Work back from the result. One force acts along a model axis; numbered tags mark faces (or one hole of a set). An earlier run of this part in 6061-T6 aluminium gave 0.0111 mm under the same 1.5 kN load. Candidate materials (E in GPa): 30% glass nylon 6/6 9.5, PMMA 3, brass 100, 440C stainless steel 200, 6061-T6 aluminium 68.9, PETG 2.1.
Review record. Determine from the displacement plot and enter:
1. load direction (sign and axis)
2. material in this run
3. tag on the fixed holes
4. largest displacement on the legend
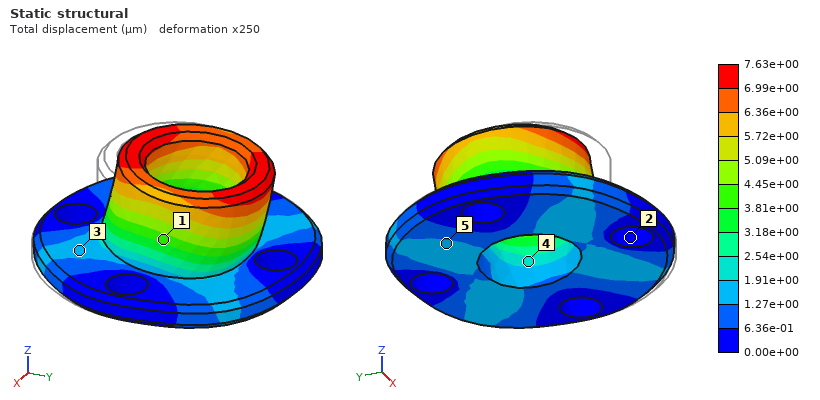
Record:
+Y
brass
2
7.63e+00 µm
